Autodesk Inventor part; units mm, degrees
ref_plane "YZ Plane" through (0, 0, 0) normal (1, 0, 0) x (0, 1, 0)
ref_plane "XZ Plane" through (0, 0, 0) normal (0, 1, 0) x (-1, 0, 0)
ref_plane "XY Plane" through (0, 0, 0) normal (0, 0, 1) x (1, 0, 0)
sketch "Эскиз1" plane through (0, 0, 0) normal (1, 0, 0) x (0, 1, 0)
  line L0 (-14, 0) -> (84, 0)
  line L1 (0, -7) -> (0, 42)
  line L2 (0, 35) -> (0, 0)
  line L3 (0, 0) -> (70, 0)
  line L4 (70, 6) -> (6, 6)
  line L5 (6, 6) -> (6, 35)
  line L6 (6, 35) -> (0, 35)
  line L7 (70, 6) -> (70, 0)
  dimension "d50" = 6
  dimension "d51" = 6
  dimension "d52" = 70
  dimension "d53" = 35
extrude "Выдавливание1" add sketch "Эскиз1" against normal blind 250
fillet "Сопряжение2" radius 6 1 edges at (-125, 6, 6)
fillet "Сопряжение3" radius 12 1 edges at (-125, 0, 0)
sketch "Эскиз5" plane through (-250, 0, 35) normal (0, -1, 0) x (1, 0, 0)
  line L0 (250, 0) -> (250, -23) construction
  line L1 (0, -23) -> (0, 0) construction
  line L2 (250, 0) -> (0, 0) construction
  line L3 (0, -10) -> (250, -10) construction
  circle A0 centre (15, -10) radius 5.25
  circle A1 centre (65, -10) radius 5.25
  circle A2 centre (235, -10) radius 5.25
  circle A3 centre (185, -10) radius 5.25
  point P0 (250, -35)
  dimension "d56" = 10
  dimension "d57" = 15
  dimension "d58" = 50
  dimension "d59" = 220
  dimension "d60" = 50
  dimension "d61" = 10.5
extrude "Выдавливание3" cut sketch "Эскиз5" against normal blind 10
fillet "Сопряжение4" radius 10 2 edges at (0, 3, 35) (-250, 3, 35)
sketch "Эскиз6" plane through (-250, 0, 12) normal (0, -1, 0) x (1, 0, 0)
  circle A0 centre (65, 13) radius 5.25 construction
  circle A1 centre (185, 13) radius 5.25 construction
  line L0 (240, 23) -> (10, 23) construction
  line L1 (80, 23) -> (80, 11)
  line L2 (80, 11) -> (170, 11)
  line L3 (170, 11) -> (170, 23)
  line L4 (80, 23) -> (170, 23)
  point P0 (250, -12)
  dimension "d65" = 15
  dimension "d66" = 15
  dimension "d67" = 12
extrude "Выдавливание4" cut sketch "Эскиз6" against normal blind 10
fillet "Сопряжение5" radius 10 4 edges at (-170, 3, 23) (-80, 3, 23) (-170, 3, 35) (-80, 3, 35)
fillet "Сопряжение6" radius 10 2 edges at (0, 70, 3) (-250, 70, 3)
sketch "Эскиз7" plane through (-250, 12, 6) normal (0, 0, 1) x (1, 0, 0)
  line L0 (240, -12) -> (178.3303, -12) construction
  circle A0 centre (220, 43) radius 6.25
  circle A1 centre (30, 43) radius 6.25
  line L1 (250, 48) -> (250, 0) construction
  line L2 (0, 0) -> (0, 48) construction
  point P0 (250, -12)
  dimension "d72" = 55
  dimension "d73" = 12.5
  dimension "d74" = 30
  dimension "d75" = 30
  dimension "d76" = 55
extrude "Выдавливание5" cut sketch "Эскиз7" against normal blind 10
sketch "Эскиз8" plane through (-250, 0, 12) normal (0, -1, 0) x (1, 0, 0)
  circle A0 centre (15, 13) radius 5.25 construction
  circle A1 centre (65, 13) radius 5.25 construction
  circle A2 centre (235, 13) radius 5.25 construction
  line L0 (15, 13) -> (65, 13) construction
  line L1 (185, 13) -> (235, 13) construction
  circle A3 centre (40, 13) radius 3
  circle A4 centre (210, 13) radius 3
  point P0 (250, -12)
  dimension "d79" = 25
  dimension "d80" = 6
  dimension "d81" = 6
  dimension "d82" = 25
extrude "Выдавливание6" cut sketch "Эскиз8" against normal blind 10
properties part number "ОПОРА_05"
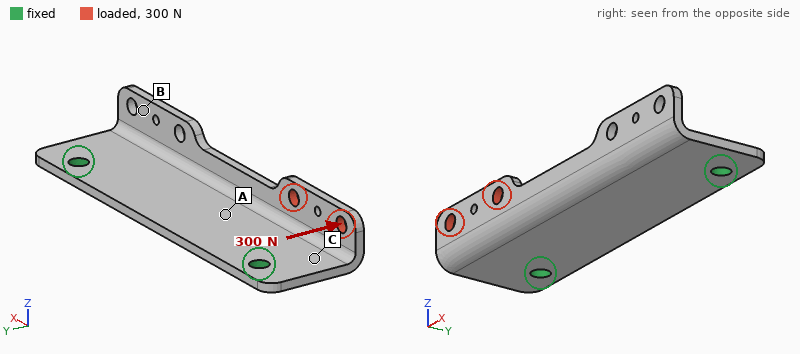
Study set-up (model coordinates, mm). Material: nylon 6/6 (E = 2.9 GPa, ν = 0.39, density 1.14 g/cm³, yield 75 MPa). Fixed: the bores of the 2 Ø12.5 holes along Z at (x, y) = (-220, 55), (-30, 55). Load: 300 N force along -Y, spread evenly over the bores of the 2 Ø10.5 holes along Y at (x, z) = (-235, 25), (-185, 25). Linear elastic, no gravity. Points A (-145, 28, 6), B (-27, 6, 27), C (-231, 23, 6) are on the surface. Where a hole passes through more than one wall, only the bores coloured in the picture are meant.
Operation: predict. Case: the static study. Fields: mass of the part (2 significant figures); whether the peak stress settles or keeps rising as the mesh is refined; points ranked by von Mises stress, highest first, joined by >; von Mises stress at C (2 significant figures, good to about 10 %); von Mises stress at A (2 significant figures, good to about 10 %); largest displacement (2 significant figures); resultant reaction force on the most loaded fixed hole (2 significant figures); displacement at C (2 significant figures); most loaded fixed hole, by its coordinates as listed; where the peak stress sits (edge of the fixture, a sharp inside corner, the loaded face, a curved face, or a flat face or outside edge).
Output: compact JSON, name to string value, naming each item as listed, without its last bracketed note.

{"mass of the part": "150 g", "whether the peak stress settles or keeps rising as the mesh is refined": "keeps rising", "points ranked by von Mises stress, highest first, joined by >": "C > A > B", "von Mises stress at C": "11 MPa", "von Mises stress at A": "2.9 MPa", "largest displacement": "3.0 mm", "resultant reaction force on the most loaded fixed hole": "290 N", "displacement at C": "0.65 mm", "most loaded fixed hole, by its coordinates as listed": "(-220, 55)", "where the peak stress sits": "edge of the fixture"}
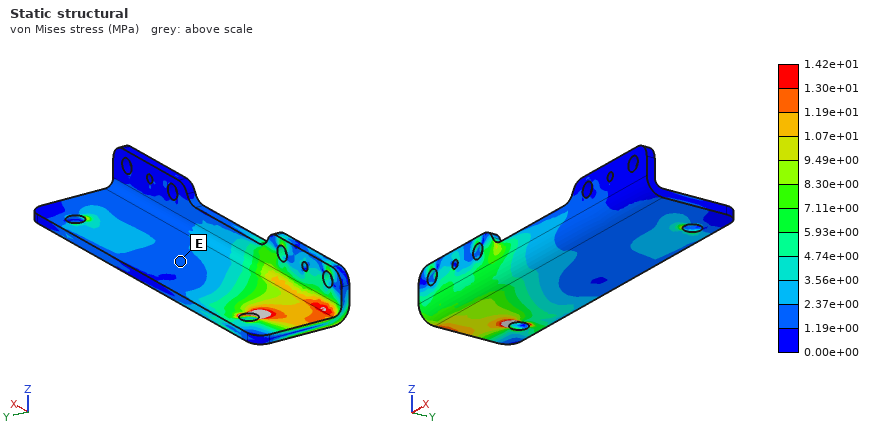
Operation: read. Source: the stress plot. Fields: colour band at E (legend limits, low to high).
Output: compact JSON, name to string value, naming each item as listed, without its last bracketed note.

{"colour band at E": "1.19e+00 to 2.37e+00 MPa"}
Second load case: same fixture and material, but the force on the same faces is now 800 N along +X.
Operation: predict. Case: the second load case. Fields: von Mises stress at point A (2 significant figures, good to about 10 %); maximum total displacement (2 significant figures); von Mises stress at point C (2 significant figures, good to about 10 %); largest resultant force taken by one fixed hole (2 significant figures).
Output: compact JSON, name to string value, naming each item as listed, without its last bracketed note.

{"von Mises stress at point A": "2.9 MPa", "maximum total displacement": "1.6 mm", "von Mises stress at point C": "4.5 MPa", "largest resultant force taken by one fixed hole": "460 N"}
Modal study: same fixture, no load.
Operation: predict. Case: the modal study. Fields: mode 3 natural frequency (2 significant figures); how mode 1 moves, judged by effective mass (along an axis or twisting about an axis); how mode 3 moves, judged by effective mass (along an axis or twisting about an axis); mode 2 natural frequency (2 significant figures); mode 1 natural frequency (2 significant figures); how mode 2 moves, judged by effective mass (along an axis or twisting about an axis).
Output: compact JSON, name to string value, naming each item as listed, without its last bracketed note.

{"mode 3 natural frequency": "380 Hz", "how mode 1 moves, judged by effective mass": "along Z", "how mode 3 moves, judged by effective mass": "along Z", "mode 2 natural frequency": "370 Hz", "mode 1 natural frequency": "240 Hz", "how mode 2 moves, judged by effective mass": "twisting about Y"}
